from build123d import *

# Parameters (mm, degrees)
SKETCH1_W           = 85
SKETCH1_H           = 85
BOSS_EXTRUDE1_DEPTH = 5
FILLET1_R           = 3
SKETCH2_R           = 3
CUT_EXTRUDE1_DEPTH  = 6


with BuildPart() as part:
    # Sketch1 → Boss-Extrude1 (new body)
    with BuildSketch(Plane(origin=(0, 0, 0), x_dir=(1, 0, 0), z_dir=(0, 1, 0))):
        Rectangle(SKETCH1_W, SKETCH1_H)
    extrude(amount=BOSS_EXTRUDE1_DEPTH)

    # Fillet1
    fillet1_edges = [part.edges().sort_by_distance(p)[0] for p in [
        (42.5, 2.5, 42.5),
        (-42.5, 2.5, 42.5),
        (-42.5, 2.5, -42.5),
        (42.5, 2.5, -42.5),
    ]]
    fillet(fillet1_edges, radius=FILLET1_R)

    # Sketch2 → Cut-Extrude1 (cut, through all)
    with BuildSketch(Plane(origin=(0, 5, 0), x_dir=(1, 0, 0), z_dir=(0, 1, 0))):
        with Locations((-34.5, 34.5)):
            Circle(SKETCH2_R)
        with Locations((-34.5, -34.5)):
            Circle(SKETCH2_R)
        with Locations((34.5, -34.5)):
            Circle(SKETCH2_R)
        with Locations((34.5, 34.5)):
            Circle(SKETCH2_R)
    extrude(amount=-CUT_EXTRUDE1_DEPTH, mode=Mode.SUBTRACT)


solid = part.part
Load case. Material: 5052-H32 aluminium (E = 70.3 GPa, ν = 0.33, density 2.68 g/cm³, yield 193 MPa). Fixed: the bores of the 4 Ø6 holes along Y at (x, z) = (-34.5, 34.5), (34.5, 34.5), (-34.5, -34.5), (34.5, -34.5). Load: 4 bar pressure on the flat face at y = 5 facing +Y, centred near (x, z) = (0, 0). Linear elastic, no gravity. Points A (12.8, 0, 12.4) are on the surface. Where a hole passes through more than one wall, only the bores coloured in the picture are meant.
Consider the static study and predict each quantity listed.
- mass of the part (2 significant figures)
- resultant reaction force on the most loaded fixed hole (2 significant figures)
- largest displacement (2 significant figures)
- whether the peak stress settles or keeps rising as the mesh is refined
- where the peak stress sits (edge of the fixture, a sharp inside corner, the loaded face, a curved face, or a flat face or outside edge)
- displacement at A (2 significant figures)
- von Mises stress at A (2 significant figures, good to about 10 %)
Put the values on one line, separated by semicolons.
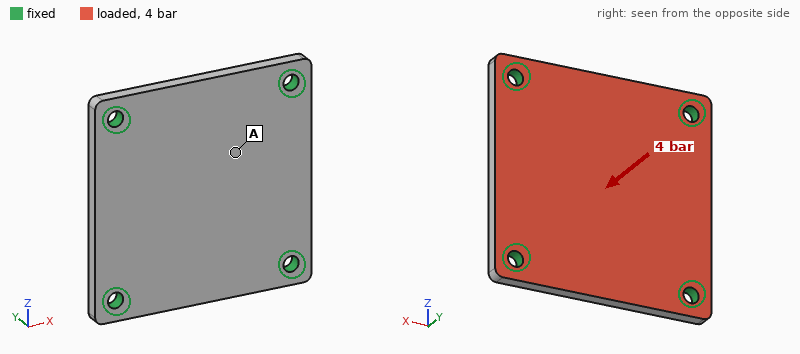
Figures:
95 g; 710 N; 77 µm; keeps rising; edge of the fixture; 63 µm; 18 MPa
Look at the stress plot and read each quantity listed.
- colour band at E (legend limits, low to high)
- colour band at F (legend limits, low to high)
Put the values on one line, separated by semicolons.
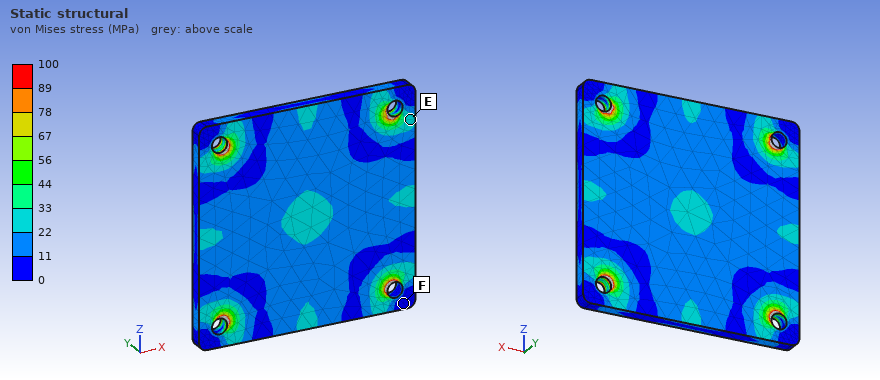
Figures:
22 to 33 MPa; 0 to 11 MPa
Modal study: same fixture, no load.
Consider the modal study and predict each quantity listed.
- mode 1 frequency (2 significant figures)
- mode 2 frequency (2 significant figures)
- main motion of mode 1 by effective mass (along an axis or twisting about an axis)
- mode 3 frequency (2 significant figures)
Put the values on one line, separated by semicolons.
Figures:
3800 Hz; 6300 Hz; along Y; 6300 Hz
